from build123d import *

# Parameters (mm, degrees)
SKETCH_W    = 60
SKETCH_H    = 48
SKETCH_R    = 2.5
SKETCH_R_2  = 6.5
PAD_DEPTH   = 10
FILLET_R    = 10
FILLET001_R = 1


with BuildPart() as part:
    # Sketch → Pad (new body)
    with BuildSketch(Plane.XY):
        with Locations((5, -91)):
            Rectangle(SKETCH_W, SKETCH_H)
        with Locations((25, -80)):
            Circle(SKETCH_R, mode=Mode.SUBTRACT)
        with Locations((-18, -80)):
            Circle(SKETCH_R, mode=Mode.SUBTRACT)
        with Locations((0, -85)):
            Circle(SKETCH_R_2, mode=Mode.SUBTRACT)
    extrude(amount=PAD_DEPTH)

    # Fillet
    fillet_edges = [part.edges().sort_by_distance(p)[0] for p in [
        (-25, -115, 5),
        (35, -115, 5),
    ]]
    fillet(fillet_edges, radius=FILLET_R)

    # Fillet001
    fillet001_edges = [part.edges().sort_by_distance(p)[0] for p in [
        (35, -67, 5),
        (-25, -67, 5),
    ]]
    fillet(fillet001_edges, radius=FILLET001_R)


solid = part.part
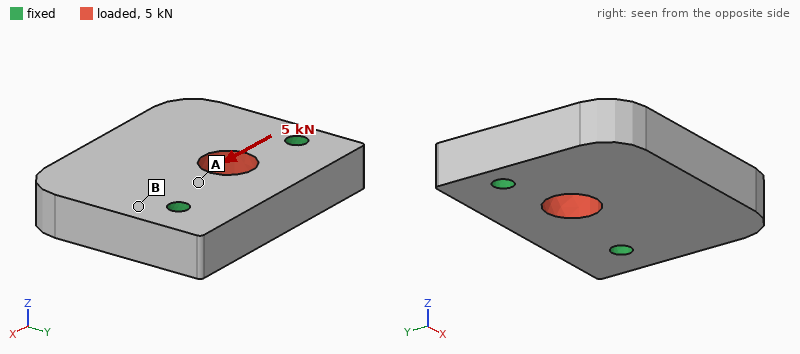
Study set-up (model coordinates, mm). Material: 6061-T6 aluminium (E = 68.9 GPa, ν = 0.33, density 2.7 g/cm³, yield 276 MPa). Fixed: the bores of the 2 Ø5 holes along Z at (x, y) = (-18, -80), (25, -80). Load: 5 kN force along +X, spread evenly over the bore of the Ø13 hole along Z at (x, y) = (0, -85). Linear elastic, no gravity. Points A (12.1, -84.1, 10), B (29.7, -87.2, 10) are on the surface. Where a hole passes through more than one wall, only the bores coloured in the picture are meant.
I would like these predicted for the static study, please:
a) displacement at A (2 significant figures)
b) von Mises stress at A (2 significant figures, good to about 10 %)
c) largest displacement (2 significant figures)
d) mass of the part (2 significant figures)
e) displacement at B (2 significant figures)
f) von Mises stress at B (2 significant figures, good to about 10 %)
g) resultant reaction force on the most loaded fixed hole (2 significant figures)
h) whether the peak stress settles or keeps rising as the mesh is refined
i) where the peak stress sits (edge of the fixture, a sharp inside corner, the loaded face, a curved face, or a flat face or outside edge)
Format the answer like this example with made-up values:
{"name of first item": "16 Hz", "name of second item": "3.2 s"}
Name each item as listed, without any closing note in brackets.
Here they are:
{"displacement at A": "3.0 µm", "von Mises stress at A": "15 MPa", "largest displacement": "5.8 µm", "mass of the part": "72 g", "displacement at B": "1.8 µm", "von Mises stress at B": "6.6 MPa", "resultant reaction force on the most loaded fixed hole": "2.7 kN", "whether the peak stress settles or keeps rising as the mesh is refined": "keeps rising", "where the peak stress sits": "edge of the fixture"}
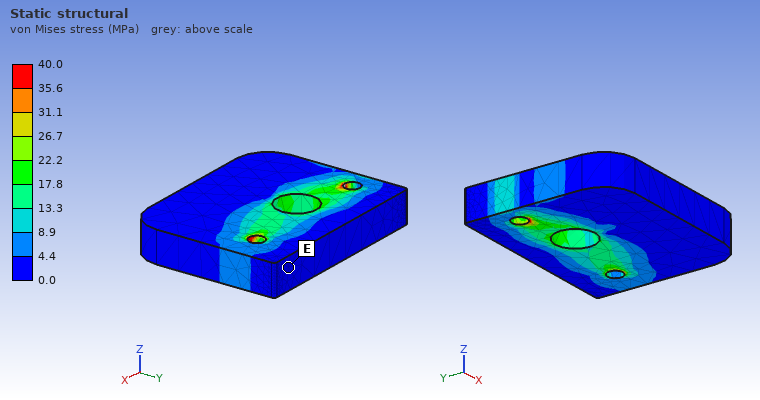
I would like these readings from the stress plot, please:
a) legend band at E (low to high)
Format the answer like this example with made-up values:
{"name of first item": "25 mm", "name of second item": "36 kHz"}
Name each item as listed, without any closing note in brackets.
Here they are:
{"legend band at E": "0.0 to 4.4 MPa"}
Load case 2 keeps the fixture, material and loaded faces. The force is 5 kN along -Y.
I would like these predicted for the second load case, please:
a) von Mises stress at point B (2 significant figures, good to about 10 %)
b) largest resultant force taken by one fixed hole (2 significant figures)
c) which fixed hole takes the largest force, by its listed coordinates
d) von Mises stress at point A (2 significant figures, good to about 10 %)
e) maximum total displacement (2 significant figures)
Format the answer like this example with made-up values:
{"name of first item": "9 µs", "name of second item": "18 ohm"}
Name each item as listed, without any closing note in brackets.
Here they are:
{"von Mises stress at point B": "5.1 MPa", "largest resultant force taken by one fixed hole": "2.9 kN", "which fixed hole takes the largest force, by its listed coordinates": "(-18, -80)", "von Mises stress at point A": "10 MPa", "maximum total displacement": "8.2 µm"}
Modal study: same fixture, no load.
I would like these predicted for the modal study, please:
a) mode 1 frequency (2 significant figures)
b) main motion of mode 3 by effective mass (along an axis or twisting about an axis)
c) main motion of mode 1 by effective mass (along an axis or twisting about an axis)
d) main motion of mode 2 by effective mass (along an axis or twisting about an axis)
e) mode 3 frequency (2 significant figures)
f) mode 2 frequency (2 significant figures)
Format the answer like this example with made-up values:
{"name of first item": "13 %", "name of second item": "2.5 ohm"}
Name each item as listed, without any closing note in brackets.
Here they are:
{"mode 1 frequency": "5300 Hz", "main motion of mode 3 by effective mass": "along X", "main motion of mode 1 by effective mass": "along Z", "main motion of mode 2 by effective mass": "twisting about Y", "mode 3 frequency": "16 kHz", "mode 2 frequency": "10 kHz"}
